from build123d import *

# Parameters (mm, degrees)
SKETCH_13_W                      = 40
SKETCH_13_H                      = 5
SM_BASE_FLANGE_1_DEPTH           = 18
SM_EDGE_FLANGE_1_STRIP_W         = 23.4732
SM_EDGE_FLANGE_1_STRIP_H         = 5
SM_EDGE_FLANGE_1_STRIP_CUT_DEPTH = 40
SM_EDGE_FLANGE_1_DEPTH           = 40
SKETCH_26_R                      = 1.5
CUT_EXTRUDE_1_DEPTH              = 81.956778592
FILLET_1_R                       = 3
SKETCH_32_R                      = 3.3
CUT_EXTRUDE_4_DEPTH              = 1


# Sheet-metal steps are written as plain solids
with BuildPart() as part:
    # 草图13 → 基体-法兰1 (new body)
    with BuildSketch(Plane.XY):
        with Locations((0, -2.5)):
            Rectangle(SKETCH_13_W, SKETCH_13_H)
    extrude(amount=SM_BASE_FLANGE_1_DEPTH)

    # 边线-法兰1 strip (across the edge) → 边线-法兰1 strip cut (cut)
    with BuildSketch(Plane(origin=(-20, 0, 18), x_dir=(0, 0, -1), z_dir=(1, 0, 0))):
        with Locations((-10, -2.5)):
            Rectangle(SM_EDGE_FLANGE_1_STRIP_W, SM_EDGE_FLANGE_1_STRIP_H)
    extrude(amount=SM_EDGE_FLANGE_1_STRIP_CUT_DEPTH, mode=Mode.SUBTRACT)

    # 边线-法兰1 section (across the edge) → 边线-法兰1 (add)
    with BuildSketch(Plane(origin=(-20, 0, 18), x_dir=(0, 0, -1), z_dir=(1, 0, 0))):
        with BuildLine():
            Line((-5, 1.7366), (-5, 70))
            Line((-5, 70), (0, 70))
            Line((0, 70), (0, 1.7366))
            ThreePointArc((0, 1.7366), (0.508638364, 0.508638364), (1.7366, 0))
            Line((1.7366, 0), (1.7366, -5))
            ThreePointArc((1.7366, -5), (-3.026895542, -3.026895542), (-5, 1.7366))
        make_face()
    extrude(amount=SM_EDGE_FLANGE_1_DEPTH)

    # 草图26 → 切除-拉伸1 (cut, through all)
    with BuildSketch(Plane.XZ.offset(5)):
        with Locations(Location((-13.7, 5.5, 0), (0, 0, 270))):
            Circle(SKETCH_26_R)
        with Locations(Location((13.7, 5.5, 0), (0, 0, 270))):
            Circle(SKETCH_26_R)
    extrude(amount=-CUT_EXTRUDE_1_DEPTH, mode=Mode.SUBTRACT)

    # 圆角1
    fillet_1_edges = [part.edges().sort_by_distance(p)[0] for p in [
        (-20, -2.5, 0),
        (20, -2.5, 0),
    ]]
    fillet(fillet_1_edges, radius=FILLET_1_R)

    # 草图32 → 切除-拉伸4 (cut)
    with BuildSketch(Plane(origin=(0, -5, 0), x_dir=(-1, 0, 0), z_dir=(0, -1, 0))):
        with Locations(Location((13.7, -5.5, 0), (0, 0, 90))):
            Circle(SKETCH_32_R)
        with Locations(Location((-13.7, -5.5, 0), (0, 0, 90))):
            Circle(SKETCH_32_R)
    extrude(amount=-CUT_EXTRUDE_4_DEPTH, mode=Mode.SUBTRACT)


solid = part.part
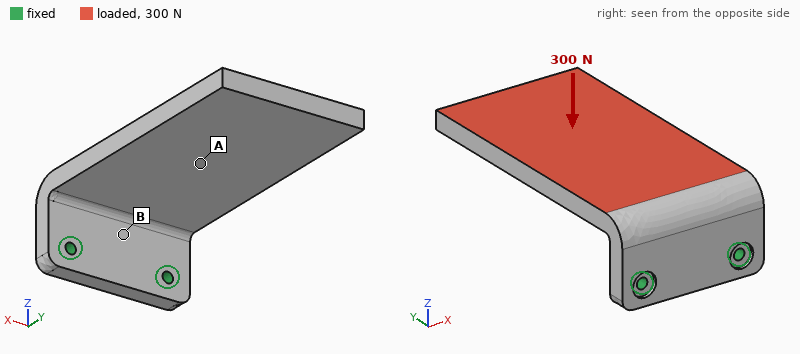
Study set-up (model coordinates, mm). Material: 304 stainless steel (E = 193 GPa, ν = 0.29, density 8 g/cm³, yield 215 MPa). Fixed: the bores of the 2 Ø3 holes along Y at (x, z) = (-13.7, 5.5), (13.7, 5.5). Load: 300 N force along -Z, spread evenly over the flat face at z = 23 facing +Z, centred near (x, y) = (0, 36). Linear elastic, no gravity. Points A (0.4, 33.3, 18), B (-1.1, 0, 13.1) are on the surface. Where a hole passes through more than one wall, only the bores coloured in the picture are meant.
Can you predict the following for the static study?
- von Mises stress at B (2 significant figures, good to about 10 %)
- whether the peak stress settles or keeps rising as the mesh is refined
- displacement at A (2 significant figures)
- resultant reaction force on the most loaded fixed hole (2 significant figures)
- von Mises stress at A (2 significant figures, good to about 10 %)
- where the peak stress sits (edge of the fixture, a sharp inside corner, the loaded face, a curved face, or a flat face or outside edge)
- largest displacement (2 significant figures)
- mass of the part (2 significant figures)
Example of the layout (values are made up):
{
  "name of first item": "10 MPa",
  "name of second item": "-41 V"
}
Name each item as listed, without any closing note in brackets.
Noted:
{
  "von Mises stress at B": "56 MPa",
  "whether the peak stress settles or keeps rising as the mesh is refined": "keeps rising",
  "displacement at A": "0.15 mm",
  "resultant reaction force on the most loaded fixed hole": "170 N",
  "von Mises stress at A": "17 MPa",
  "where the peak stress sits": "edge of the fixture",
  "largest displacement": "0.37 mm",
  "mass of the part": "140 g"
}
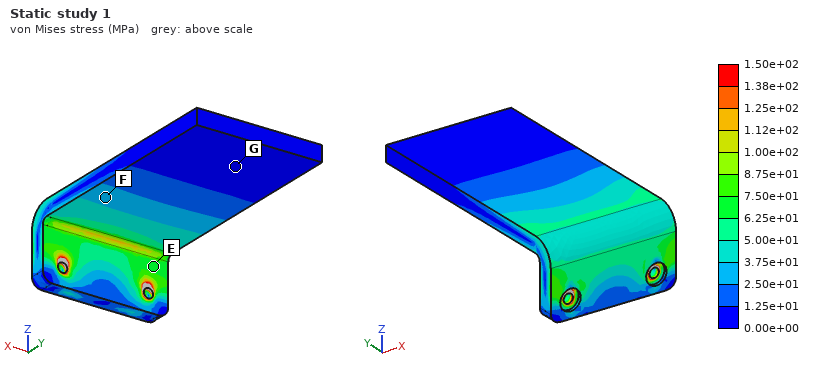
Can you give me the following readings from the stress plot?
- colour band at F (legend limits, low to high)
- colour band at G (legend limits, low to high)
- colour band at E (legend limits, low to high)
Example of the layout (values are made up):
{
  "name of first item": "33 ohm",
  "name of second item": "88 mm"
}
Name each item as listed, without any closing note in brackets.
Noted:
{
  "colour band at F": "2.50e+01 to 3.75e+01 MPa",
  "colour band at G": "0.00e+00 to 1.25e+01 MPa",
  "colour band at E": "6.25e+01 to 7.50e+01 MPa"
}
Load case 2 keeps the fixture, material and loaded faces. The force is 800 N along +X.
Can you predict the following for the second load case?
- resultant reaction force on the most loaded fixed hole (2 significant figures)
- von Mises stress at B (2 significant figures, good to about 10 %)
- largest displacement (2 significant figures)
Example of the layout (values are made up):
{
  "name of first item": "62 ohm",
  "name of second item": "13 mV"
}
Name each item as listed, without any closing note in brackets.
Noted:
{
  "resultant reaction force on the most loaded fixed hole": "1.2 kN",
  "von Mises stress at B": "76 MPa",
  "largest displacement": "0.12 mm"
}
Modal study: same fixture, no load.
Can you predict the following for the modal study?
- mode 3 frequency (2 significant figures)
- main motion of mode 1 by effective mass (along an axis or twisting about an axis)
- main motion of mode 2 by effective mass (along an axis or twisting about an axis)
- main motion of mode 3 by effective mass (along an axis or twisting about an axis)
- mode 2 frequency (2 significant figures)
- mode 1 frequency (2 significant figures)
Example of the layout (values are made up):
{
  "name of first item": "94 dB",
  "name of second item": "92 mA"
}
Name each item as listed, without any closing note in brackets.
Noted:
{
  "mode 3 frequency": "2800 Hz",
  "main motion of mode 1 by effective mass": "along Z",
  "main motion of mode 2 by effective mass": "along X",
  "main motion of mode 3 by effective mass": "twisting about Y",
  "mode 2 frequency": "1400 Hz",
  "mode 1 frequency": "540 Hz"
}
